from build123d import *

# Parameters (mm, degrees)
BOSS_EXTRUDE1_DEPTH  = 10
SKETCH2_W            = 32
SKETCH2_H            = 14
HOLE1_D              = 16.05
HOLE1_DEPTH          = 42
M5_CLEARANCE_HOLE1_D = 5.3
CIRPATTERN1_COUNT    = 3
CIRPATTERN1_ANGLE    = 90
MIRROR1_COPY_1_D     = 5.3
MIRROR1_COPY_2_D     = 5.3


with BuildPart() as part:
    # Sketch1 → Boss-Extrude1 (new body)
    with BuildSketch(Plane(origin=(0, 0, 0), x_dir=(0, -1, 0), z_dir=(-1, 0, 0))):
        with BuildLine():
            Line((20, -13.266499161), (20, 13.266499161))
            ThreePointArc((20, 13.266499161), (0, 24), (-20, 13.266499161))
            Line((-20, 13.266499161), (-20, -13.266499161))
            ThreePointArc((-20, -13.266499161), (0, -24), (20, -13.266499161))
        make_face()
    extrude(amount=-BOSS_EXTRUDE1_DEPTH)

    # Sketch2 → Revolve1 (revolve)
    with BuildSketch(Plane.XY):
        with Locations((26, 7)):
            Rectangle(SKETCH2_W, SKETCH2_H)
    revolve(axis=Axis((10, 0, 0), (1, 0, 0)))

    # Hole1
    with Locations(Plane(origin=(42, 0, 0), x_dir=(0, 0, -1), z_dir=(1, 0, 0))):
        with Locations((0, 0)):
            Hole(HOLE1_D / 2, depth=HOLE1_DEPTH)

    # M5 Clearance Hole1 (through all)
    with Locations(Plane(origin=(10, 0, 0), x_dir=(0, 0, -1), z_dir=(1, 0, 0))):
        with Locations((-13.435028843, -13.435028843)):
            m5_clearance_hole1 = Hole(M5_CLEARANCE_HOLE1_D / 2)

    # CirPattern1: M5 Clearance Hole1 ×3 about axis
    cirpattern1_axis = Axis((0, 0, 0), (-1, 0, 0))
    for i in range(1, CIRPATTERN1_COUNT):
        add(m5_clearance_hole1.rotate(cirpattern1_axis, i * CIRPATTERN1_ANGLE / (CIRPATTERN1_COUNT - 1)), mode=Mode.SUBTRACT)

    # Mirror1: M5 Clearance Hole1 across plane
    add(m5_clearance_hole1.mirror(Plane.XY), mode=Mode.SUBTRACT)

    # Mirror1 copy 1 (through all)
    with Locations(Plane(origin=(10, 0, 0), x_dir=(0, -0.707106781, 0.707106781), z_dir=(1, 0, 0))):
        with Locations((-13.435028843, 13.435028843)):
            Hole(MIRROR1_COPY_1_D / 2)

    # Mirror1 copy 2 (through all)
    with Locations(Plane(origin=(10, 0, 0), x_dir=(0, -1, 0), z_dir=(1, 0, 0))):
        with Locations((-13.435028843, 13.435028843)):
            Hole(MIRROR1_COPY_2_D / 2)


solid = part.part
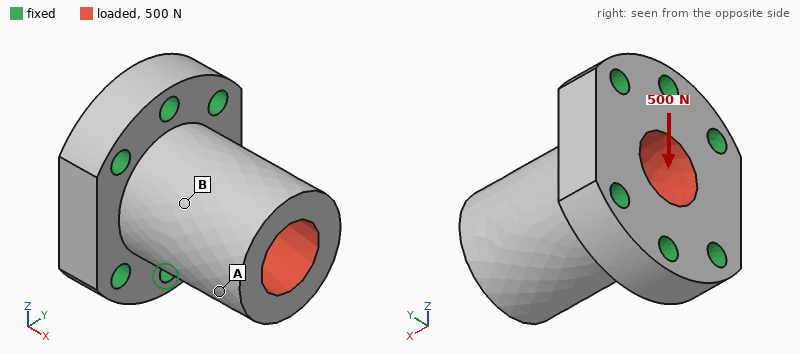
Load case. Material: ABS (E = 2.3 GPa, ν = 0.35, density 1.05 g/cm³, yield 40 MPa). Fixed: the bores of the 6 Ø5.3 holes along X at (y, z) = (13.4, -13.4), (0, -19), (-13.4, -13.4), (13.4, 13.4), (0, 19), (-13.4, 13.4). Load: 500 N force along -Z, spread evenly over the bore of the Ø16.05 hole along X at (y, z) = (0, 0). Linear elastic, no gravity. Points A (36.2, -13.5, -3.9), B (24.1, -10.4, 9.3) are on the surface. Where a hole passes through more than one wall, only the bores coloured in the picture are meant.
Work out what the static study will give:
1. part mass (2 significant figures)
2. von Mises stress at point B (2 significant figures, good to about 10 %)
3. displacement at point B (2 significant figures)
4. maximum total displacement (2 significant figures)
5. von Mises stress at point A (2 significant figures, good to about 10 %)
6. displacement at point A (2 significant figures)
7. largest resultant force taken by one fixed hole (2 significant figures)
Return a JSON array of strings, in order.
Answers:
["28 g", "1.2 MPa", "40 µm", "80 µm", "0.46 MPa", "63 µm", "160 N"]
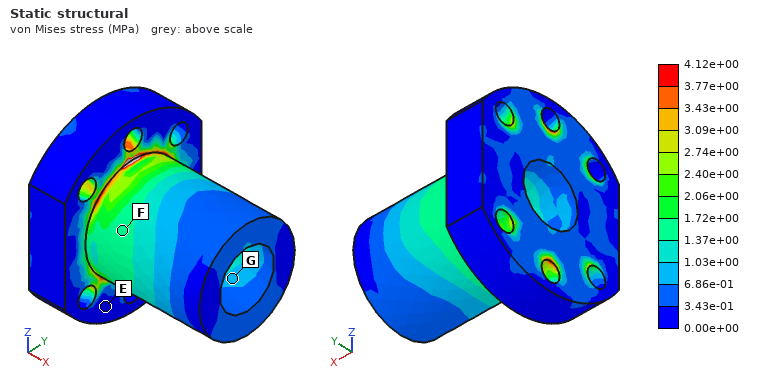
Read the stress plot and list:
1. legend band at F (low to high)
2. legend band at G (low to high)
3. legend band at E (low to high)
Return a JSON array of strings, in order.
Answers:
["1.37e+00 to 1.72e+00 MPa", "6.86e-01 to 1.03e+00 MPa", "0.00e+00 to 3.43e-01 MPa"]
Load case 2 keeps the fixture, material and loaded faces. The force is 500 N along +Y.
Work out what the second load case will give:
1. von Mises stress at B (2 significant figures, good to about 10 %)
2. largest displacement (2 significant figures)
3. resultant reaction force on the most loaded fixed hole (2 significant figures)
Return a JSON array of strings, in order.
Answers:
["1.1 MPa", "95 µm", "190 N"]
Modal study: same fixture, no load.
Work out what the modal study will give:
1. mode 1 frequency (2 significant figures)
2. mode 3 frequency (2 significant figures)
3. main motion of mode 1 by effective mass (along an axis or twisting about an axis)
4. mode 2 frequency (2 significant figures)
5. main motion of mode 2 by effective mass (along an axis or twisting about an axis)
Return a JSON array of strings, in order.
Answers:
["3200 Hz", "6400 Hz", "along Y", "3500 Hz", "along Z"]
